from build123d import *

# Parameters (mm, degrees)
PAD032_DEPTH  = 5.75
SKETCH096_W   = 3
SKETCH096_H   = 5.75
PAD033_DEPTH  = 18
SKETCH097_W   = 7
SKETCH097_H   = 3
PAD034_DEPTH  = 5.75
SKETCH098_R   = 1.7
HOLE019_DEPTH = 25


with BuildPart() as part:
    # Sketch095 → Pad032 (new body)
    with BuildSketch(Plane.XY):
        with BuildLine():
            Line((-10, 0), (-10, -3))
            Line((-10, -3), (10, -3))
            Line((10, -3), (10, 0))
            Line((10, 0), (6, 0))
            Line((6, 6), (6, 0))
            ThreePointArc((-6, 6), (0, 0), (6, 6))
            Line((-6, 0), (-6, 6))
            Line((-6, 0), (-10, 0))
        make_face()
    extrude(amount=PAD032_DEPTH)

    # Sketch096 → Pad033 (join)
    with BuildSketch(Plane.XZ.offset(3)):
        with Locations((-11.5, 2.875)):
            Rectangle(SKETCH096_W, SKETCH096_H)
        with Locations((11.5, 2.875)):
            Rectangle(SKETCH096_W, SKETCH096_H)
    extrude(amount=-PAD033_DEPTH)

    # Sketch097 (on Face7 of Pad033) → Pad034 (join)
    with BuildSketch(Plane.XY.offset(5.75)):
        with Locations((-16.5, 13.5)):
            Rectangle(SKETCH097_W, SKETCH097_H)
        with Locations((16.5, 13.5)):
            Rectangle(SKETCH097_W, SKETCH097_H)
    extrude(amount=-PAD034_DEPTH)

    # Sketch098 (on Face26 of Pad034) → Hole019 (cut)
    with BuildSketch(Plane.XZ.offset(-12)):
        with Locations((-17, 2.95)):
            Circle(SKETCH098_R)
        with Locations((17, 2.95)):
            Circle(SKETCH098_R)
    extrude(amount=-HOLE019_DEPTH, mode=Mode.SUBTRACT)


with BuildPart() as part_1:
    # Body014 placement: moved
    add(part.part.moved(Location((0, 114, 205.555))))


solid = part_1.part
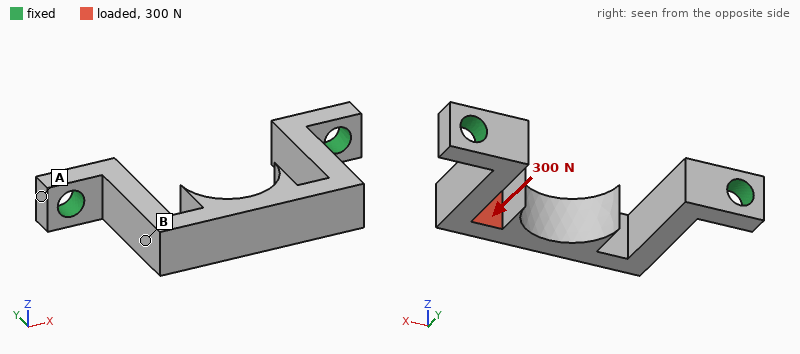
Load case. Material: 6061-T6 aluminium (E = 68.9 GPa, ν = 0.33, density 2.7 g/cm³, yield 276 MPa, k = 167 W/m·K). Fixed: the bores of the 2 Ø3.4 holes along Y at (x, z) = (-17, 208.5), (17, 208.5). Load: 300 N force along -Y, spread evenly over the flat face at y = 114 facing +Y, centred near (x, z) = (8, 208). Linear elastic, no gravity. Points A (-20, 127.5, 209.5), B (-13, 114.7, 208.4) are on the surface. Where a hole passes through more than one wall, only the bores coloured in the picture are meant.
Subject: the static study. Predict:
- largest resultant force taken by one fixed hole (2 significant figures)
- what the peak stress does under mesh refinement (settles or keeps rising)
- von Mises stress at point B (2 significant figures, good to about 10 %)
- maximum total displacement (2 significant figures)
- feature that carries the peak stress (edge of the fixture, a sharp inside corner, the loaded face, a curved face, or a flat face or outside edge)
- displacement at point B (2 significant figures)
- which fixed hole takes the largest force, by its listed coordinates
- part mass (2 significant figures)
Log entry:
260 N
keeps rising
25 MPa
26 µm
edge of the fixture
14 µm
(17, 208.5)
3.4 g
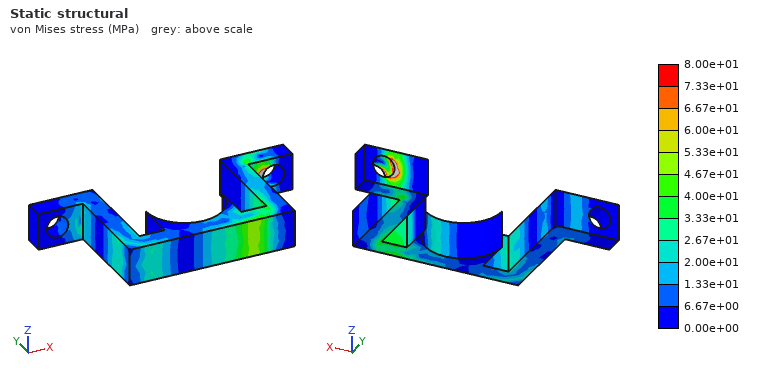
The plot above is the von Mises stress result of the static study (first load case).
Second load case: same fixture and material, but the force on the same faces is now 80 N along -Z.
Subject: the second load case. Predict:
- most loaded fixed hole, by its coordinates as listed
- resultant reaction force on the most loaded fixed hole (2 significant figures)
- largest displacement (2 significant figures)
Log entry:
(17, 208.5)
62 N
59 µm
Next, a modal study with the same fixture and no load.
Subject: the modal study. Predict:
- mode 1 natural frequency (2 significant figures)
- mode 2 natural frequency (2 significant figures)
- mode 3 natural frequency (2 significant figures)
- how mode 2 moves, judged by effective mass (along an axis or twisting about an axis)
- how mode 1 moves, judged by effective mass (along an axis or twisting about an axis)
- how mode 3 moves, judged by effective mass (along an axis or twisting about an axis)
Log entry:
5200 Hz
6600 Hz
10 kHz
along X
along Z
twisting about Y
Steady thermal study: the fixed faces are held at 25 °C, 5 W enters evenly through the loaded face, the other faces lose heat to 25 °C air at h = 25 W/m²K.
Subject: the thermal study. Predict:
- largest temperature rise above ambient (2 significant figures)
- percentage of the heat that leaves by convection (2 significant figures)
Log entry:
21 K
6.5 %
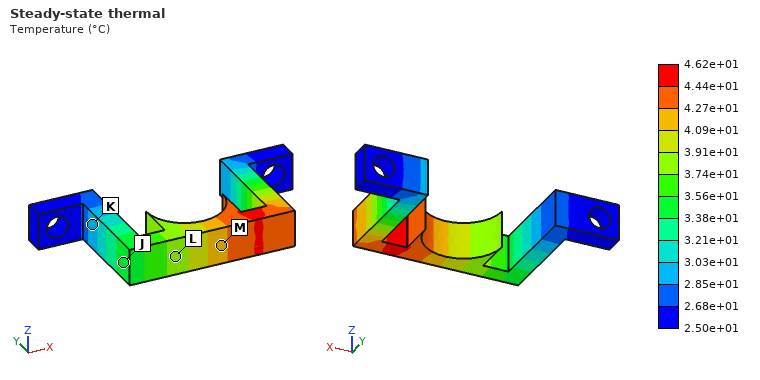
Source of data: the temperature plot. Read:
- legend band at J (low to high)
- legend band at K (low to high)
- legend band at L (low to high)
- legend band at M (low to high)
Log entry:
3.38e+01 to 3.56e+01 °C
2.85e+01 to 3.03e+01 °C
3.74e+01 to 3.91e+01 °C
4.09e+01 to 4.27e+01 °C
